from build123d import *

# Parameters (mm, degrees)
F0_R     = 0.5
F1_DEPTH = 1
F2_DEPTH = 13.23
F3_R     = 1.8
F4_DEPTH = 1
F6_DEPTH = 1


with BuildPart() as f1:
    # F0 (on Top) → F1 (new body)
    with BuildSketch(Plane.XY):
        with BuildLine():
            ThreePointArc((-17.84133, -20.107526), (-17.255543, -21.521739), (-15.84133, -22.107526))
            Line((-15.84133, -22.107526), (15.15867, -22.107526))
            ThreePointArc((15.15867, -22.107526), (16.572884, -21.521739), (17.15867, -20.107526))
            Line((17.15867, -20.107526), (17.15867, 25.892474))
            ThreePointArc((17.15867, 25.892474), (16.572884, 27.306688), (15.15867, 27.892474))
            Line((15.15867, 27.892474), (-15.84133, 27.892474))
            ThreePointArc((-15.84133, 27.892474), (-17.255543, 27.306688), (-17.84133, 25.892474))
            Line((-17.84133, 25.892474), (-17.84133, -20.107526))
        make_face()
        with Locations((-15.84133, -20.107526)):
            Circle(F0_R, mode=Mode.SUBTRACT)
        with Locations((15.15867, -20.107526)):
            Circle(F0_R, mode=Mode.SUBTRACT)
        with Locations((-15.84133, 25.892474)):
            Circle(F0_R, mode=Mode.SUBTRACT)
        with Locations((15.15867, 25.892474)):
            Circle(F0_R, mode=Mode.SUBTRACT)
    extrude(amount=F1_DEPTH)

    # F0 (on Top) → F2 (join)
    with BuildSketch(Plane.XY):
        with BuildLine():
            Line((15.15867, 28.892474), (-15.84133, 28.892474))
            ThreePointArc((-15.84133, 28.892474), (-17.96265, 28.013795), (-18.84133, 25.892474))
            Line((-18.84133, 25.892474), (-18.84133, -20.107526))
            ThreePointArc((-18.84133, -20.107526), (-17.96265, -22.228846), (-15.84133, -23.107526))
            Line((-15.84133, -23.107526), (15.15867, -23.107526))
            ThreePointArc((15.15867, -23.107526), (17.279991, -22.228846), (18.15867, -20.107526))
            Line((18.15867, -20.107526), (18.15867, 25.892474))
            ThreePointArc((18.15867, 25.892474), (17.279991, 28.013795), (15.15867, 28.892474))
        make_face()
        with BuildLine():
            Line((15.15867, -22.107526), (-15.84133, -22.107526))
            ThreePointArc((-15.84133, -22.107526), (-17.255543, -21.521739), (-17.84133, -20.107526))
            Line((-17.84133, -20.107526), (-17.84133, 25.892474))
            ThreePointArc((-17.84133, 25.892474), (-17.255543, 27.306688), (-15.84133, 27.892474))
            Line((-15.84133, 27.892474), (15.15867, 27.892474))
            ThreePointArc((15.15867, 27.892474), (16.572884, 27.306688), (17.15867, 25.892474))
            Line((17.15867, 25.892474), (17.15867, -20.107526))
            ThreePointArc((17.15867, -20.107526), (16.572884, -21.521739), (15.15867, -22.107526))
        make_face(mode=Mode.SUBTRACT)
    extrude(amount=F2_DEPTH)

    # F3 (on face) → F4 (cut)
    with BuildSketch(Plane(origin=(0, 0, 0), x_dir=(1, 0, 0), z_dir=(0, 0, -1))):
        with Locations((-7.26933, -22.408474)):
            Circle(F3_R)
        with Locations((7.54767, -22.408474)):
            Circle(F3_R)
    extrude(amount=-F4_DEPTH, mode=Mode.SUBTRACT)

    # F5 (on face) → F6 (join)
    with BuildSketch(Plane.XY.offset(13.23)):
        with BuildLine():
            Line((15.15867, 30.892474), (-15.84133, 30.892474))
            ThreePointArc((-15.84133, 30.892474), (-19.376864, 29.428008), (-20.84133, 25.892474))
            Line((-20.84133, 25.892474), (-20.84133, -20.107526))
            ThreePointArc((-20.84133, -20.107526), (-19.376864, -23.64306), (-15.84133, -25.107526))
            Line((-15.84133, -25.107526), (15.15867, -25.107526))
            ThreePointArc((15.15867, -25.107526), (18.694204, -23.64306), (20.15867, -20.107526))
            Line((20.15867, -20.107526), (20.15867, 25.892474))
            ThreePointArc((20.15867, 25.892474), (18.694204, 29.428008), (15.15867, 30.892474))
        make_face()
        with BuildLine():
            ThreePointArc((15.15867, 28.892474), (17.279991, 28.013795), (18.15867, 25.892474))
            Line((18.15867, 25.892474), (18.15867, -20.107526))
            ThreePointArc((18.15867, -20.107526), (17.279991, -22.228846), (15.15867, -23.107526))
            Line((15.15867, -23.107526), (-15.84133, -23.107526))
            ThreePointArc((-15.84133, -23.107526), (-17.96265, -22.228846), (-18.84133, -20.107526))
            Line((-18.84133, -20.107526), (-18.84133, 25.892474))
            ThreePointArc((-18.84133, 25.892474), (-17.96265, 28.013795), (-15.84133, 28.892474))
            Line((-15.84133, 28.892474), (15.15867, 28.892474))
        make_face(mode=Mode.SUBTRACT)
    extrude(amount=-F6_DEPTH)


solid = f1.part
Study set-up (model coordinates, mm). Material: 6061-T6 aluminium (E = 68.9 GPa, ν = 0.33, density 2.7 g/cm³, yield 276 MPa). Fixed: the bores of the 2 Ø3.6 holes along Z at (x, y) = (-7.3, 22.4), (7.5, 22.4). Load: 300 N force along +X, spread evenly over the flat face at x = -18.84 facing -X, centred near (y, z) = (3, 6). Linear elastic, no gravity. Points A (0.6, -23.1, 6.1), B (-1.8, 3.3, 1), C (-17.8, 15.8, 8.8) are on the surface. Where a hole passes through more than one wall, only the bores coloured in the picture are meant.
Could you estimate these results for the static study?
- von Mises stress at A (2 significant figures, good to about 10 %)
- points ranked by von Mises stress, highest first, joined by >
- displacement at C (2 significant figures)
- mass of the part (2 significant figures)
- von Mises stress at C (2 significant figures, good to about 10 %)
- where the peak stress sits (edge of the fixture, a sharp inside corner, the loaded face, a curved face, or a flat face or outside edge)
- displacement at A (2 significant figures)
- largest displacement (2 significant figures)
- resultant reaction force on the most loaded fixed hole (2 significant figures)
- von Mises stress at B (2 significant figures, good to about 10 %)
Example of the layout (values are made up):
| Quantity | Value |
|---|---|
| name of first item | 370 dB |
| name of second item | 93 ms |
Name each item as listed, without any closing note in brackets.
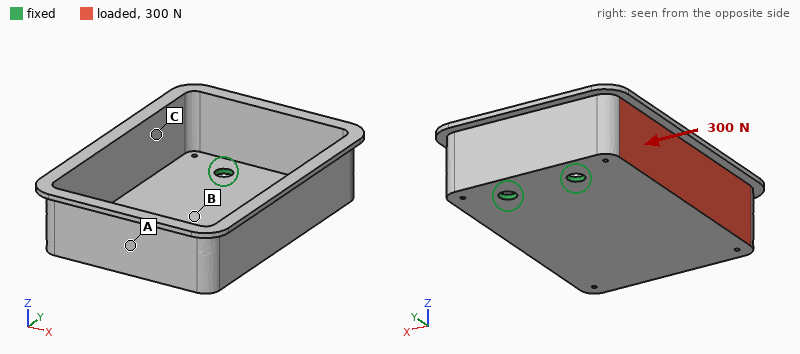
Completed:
| Quantity | Value |
|---|---|
| von Mises stress at A | 19 MPa |
| points ranked by von Mises stress, highest first, joined by > | C > B > A |
| displacement at C | 0.21 mm |
| mass of the part | 12 g |
| von Mises stress at C | 62 MPa |
| where the peak stress sits | a curved face |
| displacement at A | 0.18 mm |
| largest displacement | 0.65 mm |
| resultant reaction force on the most loaded fixed hole | 370 N |
| von Mises stress at B | 39 MPa |
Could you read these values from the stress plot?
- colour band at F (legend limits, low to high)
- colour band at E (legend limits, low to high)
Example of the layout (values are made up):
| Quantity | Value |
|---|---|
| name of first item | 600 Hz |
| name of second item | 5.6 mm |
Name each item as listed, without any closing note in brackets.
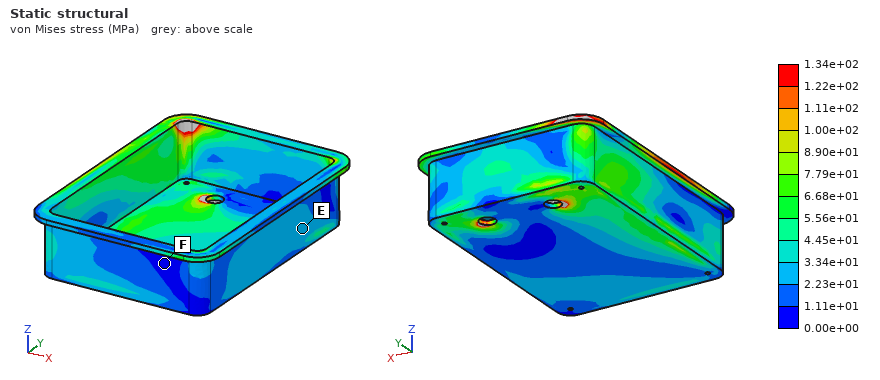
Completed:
| Quantity | Value |
|---|---|
| colour band at F | 0.00e+00 to 1.11e+01 MPa |
| colour band at E | 2.23e+01 to 3.34e+01 MPa |
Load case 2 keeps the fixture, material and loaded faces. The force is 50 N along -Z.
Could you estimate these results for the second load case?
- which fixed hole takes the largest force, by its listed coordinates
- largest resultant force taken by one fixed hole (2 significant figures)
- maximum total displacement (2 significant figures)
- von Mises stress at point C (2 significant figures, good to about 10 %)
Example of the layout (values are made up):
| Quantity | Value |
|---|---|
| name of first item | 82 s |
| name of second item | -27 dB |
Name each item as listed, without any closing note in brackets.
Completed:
| Quantity | Value |
|---|---|
| which fixed hole takes the largest force, by its listed coordinates | (-7.3, 22.4) |
| largest resultant force taken by one fixed hole | 72 N |
| maximum total displacement | 0.80 mm |
| von Mises stress at point C | 18 MPa |
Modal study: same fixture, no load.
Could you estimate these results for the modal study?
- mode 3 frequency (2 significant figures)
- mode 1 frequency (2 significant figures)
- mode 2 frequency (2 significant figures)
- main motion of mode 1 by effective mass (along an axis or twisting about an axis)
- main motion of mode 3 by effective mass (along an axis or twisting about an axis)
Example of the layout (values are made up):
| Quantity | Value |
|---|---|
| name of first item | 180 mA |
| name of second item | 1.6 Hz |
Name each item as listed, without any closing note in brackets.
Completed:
| Quantity | Value |
|---|---|
| mode 3 frequency | 3900 Hz |
| mode 1 frequency | 520 Hz |
| mode 2 frequency | 1000 Hz |
| main motion of mode 1 by effective mass | along Z |
| main motion of mode 3 by effective mass | along X |
